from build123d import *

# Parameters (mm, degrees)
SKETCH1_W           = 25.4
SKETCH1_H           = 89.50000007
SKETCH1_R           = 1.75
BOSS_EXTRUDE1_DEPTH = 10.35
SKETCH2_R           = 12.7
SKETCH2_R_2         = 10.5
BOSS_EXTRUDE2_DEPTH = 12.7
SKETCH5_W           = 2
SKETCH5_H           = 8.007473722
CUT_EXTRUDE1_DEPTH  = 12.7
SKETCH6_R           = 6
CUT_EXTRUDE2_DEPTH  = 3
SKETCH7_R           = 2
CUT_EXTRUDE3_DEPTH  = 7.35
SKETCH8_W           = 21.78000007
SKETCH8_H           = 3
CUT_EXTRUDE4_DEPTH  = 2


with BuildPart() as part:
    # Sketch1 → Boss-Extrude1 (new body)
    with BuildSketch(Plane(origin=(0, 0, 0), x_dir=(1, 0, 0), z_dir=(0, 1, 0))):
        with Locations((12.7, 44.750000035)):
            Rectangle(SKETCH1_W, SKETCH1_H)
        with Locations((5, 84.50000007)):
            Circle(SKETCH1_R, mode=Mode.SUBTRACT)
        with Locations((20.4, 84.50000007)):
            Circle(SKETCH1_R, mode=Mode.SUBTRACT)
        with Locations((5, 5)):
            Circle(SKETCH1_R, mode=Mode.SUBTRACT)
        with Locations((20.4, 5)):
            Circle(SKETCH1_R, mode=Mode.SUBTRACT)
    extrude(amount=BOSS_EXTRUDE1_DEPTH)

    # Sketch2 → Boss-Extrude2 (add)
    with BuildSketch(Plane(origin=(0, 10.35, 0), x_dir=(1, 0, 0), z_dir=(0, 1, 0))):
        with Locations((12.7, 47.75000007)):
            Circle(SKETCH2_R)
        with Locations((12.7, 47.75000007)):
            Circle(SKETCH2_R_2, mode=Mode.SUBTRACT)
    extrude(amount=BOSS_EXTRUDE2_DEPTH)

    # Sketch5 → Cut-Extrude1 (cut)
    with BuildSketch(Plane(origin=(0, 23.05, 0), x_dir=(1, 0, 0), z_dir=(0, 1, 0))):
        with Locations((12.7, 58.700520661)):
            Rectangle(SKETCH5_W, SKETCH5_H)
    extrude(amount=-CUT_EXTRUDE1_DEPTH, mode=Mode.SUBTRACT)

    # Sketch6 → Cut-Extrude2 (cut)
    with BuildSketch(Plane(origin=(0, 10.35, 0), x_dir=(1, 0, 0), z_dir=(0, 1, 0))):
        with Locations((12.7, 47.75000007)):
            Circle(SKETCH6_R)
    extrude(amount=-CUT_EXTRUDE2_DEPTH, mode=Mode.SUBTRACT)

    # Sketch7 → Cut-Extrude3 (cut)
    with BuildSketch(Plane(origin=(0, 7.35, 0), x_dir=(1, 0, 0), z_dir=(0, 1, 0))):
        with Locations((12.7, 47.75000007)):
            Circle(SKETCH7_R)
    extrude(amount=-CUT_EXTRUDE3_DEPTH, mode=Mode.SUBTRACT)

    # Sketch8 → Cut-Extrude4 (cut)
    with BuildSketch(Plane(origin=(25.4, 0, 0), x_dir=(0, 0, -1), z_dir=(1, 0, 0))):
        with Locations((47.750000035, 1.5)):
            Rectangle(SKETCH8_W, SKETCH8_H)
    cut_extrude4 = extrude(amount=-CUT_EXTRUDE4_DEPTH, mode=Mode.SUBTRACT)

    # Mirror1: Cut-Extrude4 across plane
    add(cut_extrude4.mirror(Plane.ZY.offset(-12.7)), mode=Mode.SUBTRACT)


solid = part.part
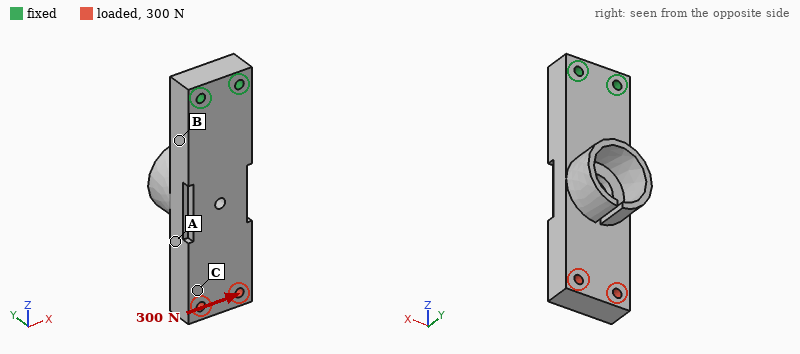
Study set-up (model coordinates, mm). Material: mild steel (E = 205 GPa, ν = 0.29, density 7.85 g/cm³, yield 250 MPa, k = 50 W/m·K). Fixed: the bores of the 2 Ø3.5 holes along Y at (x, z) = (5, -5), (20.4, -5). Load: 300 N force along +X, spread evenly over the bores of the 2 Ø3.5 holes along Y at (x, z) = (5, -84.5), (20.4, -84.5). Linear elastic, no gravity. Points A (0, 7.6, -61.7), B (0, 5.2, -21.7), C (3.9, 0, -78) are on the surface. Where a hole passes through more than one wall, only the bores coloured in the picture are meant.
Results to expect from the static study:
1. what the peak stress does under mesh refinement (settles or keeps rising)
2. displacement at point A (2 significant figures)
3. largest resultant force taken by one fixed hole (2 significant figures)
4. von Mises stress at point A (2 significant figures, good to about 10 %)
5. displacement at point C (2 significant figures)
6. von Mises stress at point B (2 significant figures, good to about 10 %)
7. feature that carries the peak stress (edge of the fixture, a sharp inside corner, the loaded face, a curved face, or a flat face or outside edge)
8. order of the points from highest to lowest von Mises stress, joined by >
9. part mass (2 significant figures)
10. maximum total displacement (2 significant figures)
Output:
keeps rising
12 µm
1.4 kN
6.6 MPa
18 µm
17 MPa
edge of the fixture
B > A > C
190 g
22 µm
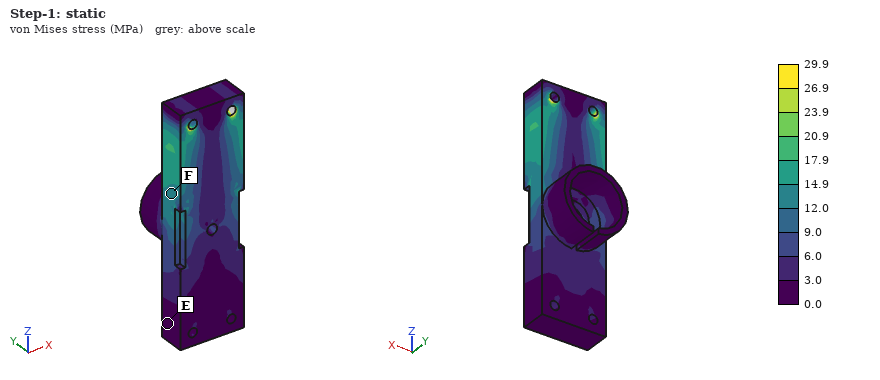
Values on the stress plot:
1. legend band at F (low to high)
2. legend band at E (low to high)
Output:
12.0 to 14.9 MPa
0.0 to 3.0 MPa
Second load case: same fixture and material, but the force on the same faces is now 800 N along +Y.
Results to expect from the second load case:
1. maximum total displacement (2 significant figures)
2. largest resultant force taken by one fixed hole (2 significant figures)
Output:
0.32 mm
400 N
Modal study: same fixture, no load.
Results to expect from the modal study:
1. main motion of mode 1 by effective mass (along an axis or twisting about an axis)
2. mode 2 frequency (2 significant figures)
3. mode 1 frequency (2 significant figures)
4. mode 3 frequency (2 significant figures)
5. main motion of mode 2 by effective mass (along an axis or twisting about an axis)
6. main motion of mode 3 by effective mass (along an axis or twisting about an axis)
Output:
along Y
2700 Hz
1200 Hz
5700 Hz
along X
twisting about Z
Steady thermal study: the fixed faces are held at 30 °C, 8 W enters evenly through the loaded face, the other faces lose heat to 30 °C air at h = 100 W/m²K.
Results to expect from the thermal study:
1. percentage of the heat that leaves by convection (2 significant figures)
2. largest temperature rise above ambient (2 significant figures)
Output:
80 %
21 K
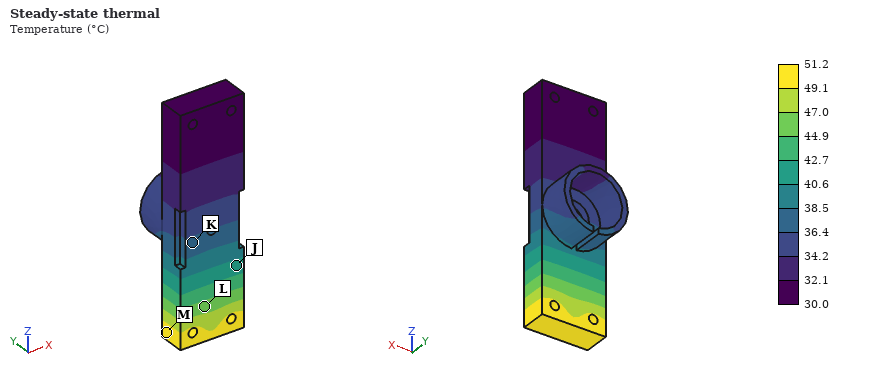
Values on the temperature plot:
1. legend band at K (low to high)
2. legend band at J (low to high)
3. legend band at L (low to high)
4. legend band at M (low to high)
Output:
36.4 to 38.5 °C
40.6 to 42.7 °C
44.9 to 47.0 °C
49.1 to 51.2 °C
